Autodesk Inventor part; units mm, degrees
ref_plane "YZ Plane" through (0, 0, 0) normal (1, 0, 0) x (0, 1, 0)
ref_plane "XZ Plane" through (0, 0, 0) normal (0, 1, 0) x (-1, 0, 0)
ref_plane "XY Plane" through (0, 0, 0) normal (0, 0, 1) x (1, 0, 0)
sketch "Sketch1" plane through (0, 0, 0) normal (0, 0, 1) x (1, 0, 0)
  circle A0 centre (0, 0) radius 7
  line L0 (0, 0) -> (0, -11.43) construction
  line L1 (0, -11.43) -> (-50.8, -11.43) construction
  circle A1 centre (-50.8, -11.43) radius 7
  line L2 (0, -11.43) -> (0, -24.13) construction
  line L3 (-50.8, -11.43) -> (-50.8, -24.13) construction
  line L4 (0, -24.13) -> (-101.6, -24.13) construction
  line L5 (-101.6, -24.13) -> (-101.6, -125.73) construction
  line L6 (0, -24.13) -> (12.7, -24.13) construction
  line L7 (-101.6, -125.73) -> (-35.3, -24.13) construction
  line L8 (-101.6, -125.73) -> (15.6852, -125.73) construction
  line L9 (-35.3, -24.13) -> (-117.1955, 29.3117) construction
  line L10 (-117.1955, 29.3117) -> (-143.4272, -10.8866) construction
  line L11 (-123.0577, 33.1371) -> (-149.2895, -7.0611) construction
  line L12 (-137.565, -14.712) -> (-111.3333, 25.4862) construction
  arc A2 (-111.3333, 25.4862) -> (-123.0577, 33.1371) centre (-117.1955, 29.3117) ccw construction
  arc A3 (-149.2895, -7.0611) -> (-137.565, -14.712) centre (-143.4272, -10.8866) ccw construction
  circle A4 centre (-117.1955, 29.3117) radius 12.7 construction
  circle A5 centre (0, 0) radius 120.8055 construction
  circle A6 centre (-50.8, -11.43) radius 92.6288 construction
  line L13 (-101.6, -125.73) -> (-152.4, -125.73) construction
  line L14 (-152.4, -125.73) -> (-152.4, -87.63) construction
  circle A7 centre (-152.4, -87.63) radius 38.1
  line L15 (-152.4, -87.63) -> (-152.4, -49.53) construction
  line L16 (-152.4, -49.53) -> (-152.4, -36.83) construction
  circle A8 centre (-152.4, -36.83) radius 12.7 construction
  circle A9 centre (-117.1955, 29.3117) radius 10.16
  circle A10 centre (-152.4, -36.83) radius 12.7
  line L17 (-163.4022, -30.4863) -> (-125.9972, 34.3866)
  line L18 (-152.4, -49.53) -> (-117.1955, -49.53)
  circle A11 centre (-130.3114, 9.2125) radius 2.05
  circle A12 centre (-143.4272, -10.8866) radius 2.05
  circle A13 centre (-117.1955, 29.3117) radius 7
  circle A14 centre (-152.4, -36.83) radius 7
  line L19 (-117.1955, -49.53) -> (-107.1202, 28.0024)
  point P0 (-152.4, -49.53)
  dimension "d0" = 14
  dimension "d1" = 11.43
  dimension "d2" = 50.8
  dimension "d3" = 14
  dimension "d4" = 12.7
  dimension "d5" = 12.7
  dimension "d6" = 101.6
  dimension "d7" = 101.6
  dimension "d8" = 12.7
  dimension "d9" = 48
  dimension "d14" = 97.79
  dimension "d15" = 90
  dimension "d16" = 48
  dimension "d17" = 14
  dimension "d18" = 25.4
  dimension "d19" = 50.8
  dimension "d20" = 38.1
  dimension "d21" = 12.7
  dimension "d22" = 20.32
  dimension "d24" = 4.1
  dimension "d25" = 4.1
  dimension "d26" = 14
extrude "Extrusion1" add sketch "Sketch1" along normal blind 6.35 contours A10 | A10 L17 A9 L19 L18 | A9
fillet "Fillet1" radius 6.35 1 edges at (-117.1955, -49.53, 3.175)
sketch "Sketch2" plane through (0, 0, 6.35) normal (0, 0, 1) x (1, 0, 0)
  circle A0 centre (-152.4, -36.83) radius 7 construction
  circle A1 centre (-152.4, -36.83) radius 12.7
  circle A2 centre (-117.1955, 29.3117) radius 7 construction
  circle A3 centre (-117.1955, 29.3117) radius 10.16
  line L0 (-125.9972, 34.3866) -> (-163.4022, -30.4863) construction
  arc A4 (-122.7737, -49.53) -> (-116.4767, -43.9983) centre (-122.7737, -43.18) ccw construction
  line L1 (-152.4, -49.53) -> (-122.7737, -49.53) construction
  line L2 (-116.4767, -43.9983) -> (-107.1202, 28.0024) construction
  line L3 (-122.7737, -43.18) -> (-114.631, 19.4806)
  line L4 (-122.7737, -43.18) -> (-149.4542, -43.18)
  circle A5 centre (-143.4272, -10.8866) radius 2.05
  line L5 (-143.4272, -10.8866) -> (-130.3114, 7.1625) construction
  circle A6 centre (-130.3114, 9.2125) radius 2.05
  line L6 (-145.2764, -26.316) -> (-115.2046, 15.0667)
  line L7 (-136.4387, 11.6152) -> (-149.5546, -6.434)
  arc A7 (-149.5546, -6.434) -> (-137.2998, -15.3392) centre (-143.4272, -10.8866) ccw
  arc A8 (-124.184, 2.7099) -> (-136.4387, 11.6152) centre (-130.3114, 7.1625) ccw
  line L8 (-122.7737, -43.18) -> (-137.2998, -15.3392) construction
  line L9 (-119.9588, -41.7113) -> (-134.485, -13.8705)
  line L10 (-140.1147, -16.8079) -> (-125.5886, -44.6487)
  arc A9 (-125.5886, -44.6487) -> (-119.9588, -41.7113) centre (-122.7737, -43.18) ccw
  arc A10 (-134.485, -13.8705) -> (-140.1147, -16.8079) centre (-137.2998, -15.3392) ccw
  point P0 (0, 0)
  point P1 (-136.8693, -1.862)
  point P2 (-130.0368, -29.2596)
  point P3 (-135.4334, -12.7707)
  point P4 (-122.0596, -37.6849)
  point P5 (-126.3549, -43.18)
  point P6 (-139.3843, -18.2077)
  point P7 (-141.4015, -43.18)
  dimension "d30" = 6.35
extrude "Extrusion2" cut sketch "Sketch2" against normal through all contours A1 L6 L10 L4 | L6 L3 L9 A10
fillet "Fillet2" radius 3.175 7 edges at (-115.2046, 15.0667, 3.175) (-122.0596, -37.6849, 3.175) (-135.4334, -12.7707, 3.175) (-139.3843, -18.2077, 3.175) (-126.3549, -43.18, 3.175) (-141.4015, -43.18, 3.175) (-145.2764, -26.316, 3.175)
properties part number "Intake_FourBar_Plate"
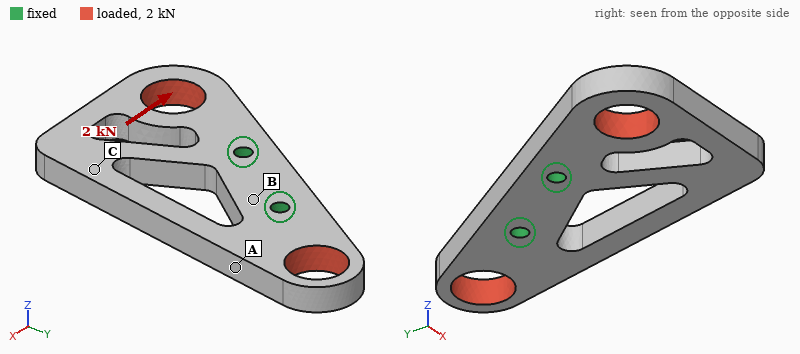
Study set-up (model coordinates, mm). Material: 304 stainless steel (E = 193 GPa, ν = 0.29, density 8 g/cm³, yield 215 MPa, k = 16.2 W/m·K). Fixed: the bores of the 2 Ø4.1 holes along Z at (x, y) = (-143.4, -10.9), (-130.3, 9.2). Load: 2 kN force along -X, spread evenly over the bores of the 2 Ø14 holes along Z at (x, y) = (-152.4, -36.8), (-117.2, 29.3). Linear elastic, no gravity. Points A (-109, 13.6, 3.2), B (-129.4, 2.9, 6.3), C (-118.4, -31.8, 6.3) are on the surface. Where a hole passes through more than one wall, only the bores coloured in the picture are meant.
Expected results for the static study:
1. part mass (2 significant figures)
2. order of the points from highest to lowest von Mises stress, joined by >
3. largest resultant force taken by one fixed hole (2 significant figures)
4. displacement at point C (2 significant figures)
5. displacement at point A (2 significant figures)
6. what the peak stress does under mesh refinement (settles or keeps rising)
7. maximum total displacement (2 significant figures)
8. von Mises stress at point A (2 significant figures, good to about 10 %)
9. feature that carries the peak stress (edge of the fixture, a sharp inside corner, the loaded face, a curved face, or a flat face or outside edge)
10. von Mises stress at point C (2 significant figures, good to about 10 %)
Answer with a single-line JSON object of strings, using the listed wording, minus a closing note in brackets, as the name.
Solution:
{"part mass": "110 g", "order of the points from highest to lowest von Mises stress, joined by >": "A > C > B", "largest resultant force taken by one fixed hole": "1.2 kN", "displacement at point C": "5.1 µm", "displacement at point A": "3.7 µm", "what the peak stress does under mesh refinement": "keeps rising", "maximum total displacement": "16 µm", "von Mises stress at point A": "25 MPa", "feature that carries the peak stress": "edge of the fixture", "von Mises stress at point C": "16 MPa"}
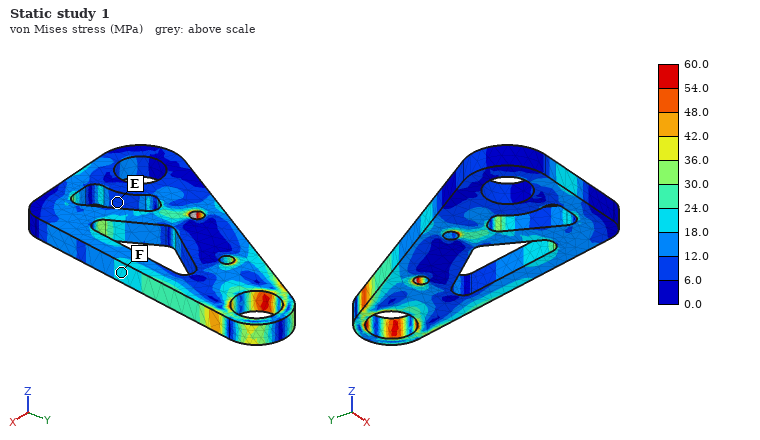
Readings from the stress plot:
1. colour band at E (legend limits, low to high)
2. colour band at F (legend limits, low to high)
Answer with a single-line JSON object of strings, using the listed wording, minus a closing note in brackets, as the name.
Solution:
{"colour band at E": "6.0 to 12.0 MPa", "colour band at F": "18.0 to 24.0 MPa"}
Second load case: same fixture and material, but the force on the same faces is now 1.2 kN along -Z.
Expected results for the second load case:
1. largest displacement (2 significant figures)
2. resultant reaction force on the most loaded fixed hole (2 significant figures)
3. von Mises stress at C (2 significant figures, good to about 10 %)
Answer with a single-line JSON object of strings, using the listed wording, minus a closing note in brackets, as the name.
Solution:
{"largest displacement": "92 µm", "resultant reaction force on the most loaded fixed hole": "620 N", "von Mises stress at C": "34 MPa"}
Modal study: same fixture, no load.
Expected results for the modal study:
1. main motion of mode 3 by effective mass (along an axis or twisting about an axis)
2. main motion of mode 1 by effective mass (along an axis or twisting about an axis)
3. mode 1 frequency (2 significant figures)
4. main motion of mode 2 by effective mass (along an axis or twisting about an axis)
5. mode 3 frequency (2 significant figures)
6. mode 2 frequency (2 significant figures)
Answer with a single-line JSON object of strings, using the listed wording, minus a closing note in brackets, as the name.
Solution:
{"main motion of mode 3 by effective mass": "along X", "main motion of mode 1 by effective mass": "along Z", "mode 1 frequency": "2300 Hz", "main motion of mode 2 by effective mass": "twisting about Y", "mode 3 frequency": "5500 Hz", "mode 2 frequency": "3800 Hz"}
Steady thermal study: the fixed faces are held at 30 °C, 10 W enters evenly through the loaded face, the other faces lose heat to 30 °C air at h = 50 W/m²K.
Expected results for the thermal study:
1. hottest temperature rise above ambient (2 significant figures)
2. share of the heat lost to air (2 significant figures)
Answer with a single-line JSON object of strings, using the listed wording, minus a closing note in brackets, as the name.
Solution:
{"hottest temperature rise above ambient": "56 K", "share of the heat lost to air": "55 %"}
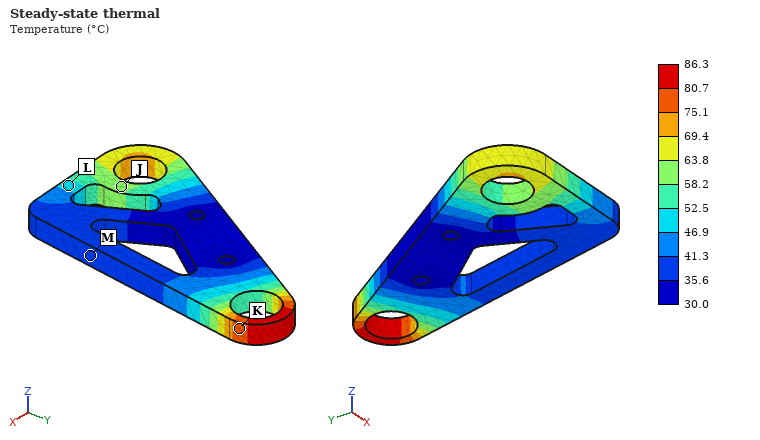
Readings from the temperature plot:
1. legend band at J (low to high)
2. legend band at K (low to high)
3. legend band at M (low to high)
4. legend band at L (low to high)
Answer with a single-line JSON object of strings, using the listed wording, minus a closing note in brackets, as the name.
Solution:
{"legend band at J": "58.2 to 63.8 °C", "legend band at K": "75.1 to 80.7 °C", "legend band at M": "35.6 to 41.3 °C", "legend band at L": "46.9 to 52.5 °C"}
